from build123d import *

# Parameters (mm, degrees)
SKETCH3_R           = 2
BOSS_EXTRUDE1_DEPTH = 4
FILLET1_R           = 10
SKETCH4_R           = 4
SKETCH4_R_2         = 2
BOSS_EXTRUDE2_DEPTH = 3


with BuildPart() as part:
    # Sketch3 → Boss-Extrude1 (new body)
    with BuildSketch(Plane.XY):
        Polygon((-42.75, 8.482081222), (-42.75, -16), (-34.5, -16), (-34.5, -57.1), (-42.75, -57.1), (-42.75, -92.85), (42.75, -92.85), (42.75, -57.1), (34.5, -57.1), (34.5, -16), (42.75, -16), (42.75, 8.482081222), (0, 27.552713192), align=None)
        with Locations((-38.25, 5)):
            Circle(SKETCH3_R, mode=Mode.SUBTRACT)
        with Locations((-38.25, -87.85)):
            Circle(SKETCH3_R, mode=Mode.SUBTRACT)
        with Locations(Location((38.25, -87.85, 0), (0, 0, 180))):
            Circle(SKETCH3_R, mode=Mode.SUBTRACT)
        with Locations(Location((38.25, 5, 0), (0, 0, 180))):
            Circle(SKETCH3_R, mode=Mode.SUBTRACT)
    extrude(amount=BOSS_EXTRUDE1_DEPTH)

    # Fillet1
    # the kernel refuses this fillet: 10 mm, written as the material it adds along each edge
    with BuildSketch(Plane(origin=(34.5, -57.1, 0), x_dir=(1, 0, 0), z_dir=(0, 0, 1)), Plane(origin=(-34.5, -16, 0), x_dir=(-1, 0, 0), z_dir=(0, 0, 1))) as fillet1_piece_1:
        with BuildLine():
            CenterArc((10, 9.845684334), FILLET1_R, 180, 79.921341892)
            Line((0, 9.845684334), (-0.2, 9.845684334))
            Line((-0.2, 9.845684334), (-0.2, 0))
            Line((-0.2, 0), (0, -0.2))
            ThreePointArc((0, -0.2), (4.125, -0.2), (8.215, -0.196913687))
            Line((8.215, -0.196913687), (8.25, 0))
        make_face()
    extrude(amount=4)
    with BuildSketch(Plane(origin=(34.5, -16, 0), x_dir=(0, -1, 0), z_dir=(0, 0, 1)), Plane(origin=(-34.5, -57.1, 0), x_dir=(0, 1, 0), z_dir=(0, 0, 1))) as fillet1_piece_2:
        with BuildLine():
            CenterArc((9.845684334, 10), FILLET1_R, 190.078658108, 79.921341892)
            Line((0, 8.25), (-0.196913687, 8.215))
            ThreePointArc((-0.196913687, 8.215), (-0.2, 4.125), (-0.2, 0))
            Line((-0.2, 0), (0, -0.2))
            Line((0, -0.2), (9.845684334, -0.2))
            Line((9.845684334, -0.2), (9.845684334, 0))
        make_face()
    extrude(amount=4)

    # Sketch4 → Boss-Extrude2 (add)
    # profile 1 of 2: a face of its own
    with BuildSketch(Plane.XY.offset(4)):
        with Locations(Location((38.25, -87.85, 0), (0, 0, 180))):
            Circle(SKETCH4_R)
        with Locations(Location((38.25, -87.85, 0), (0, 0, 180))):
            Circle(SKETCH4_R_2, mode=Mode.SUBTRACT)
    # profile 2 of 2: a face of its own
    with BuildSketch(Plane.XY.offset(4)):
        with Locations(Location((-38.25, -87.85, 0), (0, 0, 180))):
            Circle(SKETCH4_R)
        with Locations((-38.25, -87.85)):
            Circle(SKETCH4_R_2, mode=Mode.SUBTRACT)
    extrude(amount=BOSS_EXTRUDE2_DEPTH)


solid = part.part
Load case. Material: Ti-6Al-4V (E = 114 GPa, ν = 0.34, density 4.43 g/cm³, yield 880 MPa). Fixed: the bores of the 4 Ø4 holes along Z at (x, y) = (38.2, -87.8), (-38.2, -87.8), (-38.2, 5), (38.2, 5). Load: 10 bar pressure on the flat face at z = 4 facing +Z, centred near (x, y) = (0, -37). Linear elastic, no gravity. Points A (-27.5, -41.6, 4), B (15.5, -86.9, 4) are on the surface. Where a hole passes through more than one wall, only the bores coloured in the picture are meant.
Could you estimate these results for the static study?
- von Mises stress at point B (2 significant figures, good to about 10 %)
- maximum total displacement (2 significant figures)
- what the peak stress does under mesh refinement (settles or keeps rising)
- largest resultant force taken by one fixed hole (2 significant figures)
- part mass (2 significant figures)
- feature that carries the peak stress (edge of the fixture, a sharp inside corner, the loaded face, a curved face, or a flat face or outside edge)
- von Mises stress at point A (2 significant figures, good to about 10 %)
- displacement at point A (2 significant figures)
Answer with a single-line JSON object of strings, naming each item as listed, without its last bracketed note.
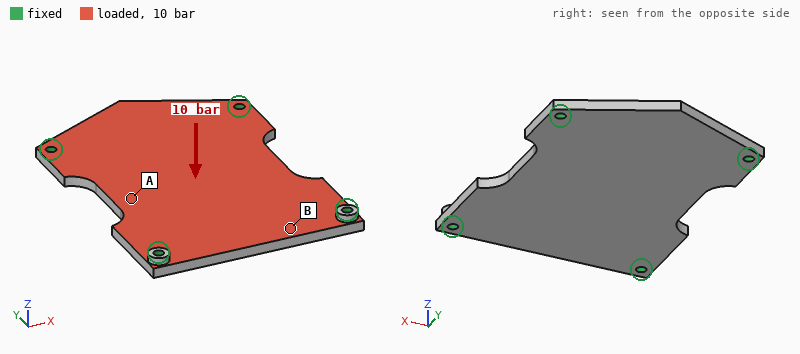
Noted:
{"von Mises stress at point B": "73 MPa", "maximum total displacement": "0.63 mm", "what the peak stress does under mesh refinement": "keeps rising", "largest resultant force taken by one fixed hole": "2.4 kN", "part mass": "160 g", "feature that carries the peak stress": "edge of the fixture", "von Mises stress at point A": "180 MPa", "displacement at point A": "0.54 mm"}
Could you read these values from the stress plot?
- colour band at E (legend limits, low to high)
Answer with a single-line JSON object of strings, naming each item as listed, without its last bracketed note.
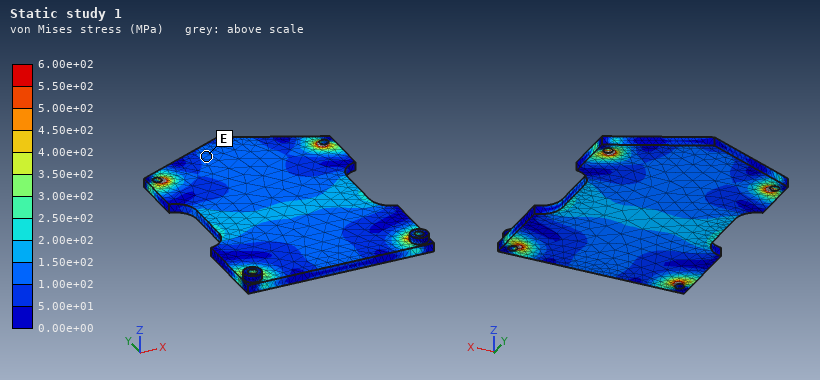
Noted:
{"colour band at E": "1.00e+02 to 1.50e+02 MPa"}
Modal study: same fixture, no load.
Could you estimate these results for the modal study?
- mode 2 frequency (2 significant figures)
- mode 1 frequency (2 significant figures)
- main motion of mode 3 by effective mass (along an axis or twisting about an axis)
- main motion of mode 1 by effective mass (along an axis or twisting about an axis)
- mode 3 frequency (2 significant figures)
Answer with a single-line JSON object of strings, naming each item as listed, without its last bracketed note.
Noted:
{"mode 2 frequency": "3000 Hz", "mode 1 frequency": "1800 Hz", "main motion of mode 3 by effective mass": "twisting about Y", "main motion of mode 1 by effective mass": "along Z", "mode 3 frequency": "3300 Hz"}
